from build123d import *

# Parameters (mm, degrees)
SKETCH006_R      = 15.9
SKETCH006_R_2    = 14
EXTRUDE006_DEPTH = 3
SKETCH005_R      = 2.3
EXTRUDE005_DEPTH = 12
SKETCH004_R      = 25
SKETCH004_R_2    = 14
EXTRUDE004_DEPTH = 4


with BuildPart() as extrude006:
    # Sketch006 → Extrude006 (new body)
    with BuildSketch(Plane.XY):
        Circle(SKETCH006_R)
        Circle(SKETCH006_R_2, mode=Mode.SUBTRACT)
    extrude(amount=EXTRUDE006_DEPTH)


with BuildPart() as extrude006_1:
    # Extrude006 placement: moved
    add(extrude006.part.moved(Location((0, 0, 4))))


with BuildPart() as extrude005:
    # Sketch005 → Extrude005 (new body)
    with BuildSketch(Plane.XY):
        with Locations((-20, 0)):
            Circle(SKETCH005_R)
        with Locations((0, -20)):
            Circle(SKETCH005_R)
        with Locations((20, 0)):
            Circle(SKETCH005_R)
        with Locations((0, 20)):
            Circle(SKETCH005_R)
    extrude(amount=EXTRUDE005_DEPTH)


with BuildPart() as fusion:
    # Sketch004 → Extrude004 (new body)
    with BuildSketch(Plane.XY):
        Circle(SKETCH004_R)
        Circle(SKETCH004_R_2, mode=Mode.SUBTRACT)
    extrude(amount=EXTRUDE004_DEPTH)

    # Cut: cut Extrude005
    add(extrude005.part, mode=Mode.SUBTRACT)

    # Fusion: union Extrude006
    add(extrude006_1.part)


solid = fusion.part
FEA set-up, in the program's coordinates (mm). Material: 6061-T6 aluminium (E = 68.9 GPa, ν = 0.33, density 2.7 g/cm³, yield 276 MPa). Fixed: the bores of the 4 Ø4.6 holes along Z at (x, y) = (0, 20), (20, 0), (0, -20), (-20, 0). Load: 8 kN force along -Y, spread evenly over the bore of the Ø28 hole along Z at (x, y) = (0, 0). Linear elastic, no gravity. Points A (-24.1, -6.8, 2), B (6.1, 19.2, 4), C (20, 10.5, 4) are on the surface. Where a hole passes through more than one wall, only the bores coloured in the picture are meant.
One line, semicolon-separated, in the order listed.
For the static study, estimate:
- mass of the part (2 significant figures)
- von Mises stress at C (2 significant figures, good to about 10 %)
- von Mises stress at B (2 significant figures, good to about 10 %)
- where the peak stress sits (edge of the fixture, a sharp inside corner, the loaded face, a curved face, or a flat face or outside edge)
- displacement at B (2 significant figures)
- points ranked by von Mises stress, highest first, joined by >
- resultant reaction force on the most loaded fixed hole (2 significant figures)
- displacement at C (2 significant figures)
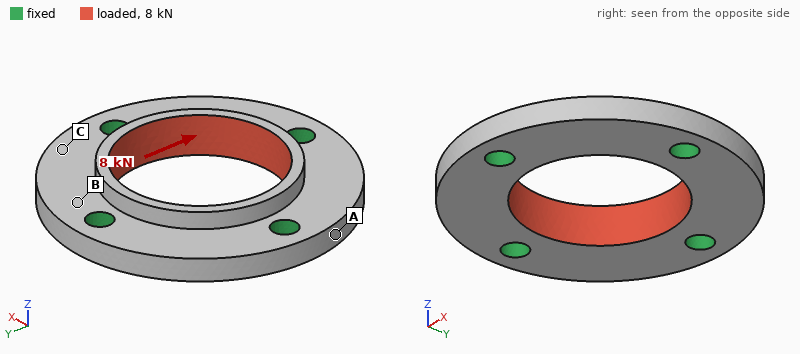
15 g; 20 MPa; 36 MPa; edge of the fixture; 4.6 µm; B > C > A; 2.3 kN; 6.4 µm
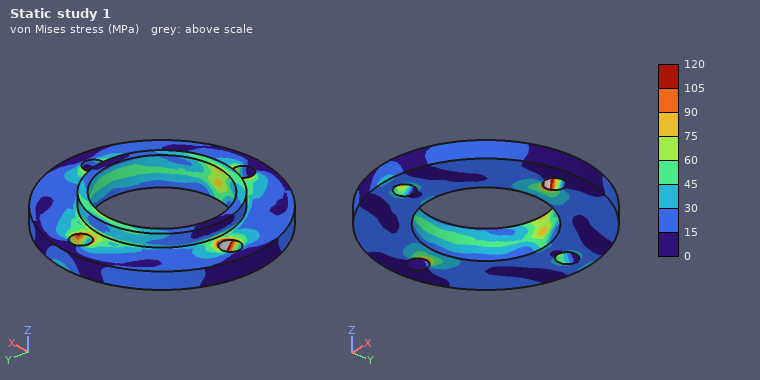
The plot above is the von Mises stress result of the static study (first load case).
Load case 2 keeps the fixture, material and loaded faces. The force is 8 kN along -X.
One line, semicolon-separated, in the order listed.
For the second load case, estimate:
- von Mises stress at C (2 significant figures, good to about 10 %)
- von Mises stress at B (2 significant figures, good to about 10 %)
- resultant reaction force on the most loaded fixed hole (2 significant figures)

17 MPa; 36 MPa; 2.3 kN
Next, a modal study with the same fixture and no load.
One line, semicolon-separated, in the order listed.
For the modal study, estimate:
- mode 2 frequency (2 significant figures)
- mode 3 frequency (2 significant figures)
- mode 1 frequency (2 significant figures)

21 kHz; 21 kHz; 20 kHz
